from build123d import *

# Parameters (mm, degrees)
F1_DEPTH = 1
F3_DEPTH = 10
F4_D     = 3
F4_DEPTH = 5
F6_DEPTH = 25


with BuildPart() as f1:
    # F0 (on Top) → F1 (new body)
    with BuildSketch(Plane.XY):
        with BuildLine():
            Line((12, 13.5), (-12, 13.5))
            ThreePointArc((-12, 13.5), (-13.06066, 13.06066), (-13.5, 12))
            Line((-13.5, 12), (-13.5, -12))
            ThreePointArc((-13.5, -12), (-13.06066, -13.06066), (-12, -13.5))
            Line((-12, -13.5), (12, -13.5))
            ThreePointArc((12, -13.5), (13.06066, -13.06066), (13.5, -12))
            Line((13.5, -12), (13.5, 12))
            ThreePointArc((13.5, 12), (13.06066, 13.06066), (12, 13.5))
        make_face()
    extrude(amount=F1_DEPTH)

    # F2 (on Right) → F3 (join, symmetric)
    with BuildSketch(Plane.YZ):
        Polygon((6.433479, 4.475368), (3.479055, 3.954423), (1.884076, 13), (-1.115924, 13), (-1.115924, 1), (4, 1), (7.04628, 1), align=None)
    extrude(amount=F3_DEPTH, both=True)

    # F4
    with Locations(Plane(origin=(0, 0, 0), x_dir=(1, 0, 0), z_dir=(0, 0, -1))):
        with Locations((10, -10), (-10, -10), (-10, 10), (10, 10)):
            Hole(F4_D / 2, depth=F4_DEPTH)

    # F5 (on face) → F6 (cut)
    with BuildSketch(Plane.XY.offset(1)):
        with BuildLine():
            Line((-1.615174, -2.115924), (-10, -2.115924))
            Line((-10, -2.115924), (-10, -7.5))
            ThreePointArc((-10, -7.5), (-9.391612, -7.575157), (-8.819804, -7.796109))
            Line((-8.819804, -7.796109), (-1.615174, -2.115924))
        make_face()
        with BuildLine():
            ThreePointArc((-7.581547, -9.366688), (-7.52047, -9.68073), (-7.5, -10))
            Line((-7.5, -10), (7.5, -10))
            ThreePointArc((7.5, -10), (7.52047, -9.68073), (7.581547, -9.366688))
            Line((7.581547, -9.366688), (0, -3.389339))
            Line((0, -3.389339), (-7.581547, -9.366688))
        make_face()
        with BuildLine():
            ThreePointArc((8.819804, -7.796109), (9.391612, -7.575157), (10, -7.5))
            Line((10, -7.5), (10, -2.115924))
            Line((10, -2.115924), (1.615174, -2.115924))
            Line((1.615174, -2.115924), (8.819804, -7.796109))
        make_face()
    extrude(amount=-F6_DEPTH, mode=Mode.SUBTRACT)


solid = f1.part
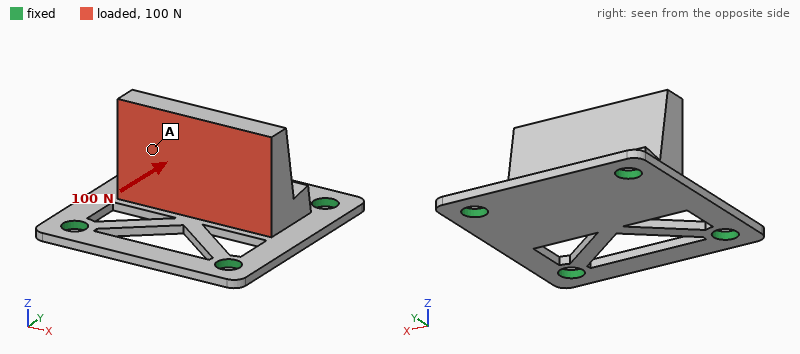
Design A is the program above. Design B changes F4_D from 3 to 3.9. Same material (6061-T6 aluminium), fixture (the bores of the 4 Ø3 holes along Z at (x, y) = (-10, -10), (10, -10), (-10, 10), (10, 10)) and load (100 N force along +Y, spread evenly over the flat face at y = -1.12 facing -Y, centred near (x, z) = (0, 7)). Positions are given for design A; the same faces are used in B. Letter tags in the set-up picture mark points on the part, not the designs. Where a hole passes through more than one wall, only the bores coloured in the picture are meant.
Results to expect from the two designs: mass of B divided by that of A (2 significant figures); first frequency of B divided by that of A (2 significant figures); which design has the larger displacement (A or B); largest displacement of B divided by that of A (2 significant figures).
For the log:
0.99
1.1
A
0.90
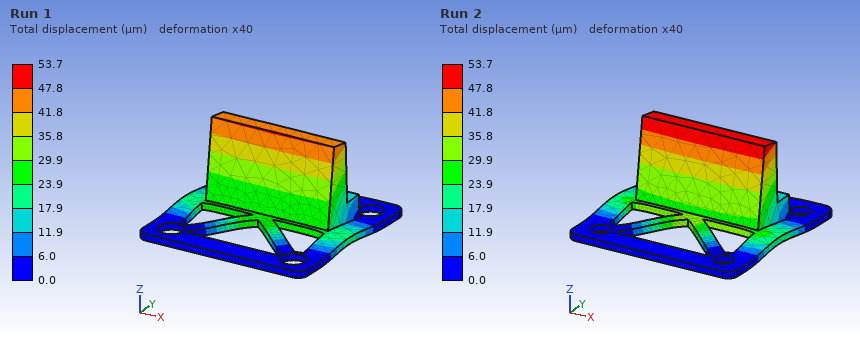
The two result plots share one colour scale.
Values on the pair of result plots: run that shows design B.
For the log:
Run 1
